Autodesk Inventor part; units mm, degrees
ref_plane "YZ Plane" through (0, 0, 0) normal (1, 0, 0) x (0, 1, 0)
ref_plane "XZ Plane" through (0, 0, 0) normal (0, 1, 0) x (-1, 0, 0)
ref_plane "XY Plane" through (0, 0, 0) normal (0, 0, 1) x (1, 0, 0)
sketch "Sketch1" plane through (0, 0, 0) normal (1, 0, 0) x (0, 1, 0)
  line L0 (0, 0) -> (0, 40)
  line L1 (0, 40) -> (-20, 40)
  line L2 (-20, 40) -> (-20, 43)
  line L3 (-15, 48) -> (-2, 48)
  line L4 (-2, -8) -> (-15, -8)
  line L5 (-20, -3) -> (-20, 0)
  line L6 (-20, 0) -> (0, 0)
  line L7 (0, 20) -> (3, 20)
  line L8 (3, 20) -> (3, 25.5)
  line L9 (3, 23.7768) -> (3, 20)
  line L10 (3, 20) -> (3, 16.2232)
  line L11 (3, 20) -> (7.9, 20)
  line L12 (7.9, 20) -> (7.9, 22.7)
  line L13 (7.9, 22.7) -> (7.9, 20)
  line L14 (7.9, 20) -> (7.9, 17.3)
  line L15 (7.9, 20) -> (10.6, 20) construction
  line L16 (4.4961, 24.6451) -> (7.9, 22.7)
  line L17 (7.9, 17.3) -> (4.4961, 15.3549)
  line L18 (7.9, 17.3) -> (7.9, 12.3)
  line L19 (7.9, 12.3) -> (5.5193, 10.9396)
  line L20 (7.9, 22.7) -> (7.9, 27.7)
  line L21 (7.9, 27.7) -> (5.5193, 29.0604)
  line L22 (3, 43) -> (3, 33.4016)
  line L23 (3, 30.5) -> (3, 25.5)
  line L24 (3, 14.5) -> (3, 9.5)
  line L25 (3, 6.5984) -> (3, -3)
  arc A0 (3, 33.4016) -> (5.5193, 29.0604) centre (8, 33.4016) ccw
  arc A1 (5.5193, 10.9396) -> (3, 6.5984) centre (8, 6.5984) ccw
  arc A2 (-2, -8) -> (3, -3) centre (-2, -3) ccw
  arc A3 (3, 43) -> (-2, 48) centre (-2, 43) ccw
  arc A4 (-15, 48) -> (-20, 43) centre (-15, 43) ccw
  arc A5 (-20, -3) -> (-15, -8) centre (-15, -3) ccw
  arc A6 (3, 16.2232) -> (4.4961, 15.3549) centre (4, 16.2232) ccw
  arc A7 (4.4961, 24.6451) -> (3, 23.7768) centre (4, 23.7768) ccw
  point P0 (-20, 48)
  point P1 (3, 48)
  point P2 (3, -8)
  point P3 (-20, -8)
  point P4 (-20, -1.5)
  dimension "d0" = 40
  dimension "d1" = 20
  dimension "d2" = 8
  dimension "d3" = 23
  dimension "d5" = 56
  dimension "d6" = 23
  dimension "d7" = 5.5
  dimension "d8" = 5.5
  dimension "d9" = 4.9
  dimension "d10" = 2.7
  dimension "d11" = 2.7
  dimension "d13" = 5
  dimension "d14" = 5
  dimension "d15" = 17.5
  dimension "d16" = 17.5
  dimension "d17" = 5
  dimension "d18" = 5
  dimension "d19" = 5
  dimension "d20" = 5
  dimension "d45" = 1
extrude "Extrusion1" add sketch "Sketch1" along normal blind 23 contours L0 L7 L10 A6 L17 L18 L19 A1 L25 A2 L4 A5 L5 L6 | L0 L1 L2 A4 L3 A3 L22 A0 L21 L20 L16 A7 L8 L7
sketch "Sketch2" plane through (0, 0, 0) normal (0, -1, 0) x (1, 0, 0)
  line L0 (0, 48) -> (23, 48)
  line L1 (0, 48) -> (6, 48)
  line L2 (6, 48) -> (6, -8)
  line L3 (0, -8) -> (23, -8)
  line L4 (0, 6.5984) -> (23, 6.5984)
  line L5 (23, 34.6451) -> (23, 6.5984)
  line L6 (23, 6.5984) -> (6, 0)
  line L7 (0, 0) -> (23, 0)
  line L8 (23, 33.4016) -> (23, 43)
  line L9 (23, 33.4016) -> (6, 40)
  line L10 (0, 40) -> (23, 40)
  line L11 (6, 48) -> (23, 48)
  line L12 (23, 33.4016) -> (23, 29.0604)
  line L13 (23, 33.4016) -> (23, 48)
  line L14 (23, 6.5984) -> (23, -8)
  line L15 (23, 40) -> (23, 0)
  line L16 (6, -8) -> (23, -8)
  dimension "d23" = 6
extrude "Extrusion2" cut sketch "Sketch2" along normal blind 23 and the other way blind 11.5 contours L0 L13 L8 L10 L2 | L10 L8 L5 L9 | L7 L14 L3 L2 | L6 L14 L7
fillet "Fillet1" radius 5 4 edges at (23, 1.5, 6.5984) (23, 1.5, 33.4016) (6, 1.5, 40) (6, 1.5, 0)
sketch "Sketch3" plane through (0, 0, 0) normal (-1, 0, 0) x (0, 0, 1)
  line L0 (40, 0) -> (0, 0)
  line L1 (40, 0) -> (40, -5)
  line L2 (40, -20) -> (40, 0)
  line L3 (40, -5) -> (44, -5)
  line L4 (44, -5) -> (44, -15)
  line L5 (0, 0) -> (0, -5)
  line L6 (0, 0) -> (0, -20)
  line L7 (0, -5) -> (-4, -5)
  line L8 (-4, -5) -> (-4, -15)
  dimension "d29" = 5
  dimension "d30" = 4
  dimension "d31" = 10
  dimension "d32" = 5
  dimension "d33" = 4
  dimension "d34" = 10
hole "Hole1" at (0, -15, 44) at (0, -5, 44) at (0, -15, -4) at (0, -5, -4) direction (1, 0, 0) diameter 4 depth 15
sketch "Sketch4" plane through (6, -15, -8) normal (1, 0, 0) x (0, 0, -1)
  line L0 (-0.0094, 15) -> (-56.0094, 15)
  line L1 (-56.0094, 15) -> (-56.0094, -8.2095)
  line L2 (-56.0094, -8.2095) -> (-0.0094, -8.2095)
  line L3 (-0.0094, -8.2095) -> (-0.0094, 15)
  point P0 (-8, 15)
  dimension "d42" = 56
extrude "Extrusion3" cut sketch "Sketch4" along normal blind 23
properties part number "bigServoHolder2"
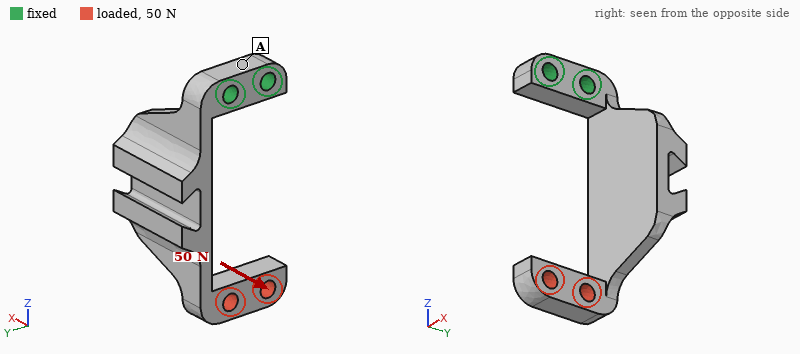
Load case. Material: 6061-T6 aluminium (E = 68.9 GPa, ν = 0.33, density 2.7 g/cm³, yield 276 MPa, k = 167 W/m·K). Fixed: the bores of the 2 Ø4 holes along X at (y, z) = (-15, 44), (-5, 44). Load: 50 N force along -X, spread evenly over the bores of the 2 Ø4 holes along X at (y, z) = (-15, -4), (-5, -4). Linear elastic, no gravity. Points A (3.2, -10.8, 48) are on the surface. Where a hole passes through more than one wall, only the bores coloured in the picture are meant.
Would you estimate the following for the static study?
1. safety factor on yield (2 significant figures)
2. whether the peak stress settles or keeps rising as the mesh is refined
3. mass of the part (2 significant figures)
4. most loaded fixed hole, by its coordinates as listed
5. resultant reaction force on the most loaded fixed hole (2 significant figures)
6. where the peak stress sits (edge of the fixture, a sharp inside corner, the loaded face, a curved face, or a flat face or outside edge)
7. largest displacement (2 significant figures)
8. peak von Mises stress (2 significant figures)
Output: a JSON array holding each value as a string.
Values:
["1.8", "settles", "15 g", "(-5, 44)", "47 N", "a curved face", "0.38 mm", "150 MPa"]
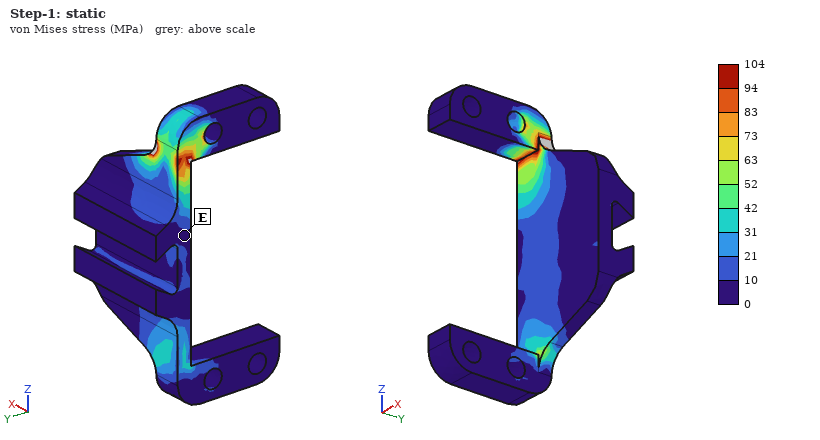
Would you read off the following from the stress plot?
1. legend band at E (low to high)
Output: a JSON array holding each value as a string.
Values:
["0 to 10 MPa"]
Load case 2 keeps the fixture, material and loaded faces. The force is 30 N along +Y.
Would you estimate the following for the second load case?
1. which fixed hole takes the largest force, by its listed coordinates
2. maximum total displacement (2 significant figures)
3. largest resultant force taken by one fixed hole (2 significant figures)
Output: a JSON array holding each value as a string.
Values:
["(-5, 44)", "0.59 mm", "41 N"]
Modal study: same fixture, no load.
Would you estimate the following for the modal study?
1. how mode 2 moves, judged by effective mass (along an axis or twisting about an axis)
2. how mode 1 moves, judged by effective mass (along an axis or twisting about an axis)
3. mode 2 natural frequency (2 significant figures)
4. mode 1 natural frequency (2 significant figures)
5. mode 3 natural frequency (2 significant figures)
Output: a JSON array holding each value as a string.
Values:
["along X", "along Y", "1100 Hz", "580 Hz", "1900 Hz"]
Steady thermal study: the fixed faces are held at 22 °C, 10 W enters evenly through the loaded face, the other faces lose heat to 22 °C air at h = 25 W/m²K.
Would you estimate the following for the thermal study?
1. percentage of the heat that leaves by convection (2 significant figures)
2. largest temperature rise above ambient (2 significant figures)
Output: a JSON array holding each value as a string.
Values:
["28 %", "75 K"]
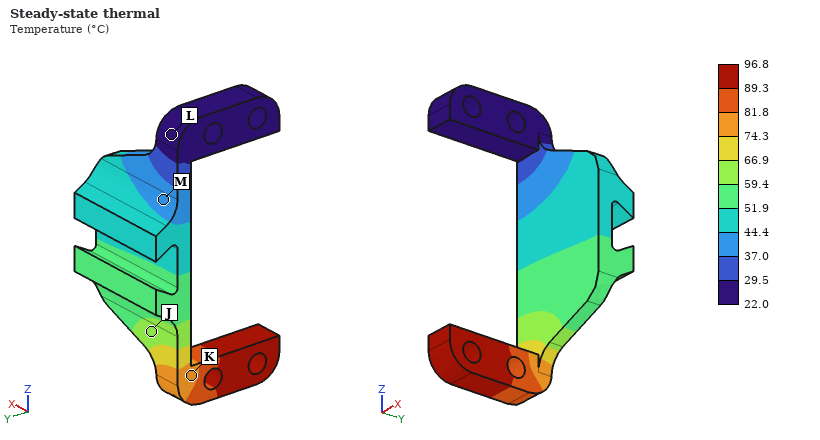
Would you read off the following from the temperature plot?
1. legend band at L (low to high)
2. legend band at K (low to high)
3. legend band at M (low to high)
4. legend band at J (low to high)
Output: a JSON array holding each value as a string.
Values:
["22.0 to 29.5 °C", "74.3 to 81.8 °C", "37.0 to 44.4 °C", "59.4 to 66.9 °C"]
